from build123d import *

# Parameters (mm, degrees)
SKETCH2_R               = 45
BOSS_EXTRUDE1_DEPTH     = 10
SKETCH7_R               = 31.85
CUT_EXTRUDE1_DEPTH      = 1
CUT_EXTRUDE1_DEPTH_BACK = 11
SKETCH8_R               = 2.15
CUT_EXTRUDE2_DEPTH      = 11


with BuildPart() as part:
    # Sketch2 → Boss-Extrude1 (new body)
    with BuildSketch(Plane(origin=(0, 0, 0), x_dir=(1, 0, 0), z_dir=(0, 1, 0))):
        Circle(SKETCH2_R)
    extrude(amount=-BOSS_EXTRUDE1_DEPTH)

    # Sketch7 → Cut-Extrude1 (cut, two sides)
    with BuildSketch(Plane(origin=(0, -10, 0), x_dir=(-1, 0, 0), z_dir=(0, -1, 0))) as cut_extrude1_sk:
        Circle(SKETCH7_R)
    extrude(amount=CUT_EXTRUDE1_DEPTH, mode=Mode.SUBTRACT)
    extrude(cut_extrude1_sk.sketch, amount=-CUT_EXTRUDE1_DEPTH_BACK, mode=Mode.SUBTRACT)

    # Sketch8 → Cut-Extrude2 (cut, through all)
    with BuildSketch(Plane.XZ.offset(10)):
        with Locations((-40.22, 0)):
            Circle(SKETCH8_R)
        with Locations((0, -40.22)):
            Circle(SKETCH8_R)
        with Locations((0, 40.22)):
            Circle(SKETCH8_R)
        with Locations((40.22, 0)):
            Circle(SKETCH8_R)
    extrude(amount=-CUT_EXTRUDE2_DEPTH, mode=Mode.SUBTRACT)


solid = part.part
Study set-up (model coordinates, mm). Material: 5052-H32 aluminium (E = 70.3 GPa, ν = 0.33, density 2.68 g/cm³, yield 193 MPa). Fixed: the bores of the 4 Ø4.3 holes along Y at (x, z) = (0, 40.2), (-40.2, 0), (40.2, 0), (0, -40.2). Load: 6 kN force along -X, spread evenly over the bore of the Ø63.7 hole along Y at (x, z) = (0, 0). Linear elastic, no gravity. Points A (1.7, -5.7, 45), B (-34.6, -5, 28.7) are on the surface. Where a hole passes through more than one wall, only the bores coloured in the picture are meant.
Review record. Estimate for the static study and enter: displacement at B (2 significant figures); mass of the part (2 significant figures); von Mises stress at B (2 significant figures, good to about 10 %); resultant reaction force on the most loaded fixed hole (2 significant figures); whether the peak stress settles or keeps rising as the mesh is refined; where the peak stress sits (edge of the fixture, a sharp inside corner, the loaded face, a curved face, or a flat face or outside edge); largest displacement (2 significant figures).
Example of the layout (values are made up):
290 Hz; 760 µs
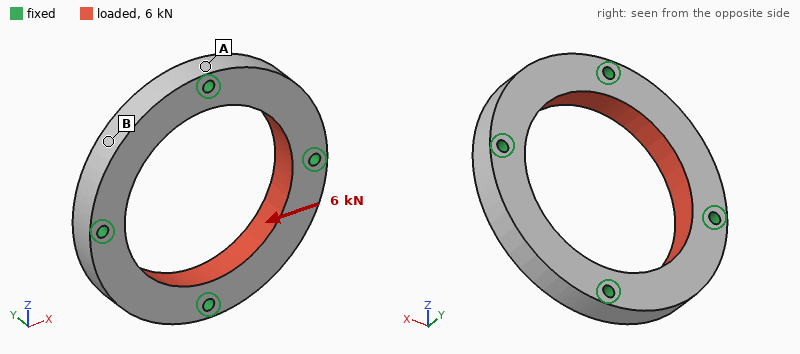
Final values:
4.7 µm; 84 g; 8.1 MPa; 2.0 kN; keeps rising; edge of the fixture; 5.2 µm
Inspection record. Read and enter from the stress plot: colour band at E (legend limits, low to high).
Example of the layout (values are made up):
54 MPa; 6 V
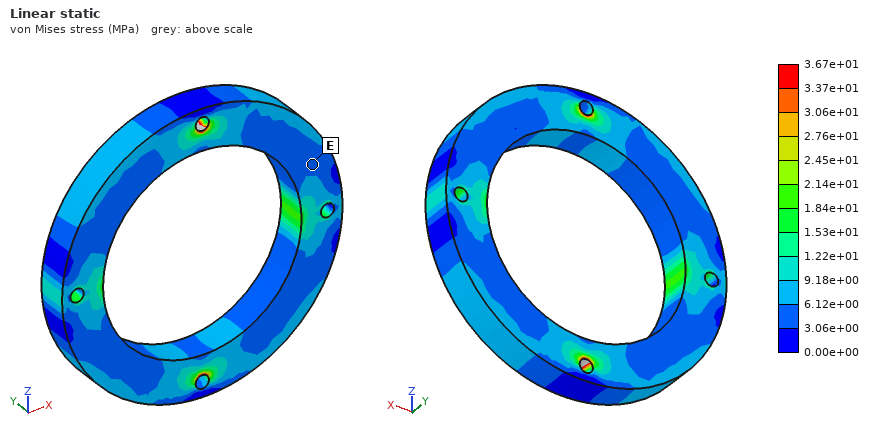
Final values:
3.06e+00 to 6.12e+00 MPa
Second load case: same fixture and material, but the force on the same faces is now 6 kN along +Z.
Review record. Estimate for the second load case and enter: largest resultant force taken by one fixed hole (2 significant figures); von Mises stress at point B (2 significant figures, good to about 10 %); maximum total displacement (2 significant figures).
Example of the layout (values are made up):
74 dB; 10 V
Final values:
2.0 kN; 7.8 MPa; 5.2 µm
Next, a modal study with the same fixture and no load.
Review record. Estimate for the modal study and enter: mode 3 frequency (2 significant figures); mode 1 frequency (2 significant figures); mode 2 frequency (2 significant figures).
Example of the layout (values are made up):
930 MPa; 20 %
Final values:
11 kHz; 11 kHz; 11 kHz
